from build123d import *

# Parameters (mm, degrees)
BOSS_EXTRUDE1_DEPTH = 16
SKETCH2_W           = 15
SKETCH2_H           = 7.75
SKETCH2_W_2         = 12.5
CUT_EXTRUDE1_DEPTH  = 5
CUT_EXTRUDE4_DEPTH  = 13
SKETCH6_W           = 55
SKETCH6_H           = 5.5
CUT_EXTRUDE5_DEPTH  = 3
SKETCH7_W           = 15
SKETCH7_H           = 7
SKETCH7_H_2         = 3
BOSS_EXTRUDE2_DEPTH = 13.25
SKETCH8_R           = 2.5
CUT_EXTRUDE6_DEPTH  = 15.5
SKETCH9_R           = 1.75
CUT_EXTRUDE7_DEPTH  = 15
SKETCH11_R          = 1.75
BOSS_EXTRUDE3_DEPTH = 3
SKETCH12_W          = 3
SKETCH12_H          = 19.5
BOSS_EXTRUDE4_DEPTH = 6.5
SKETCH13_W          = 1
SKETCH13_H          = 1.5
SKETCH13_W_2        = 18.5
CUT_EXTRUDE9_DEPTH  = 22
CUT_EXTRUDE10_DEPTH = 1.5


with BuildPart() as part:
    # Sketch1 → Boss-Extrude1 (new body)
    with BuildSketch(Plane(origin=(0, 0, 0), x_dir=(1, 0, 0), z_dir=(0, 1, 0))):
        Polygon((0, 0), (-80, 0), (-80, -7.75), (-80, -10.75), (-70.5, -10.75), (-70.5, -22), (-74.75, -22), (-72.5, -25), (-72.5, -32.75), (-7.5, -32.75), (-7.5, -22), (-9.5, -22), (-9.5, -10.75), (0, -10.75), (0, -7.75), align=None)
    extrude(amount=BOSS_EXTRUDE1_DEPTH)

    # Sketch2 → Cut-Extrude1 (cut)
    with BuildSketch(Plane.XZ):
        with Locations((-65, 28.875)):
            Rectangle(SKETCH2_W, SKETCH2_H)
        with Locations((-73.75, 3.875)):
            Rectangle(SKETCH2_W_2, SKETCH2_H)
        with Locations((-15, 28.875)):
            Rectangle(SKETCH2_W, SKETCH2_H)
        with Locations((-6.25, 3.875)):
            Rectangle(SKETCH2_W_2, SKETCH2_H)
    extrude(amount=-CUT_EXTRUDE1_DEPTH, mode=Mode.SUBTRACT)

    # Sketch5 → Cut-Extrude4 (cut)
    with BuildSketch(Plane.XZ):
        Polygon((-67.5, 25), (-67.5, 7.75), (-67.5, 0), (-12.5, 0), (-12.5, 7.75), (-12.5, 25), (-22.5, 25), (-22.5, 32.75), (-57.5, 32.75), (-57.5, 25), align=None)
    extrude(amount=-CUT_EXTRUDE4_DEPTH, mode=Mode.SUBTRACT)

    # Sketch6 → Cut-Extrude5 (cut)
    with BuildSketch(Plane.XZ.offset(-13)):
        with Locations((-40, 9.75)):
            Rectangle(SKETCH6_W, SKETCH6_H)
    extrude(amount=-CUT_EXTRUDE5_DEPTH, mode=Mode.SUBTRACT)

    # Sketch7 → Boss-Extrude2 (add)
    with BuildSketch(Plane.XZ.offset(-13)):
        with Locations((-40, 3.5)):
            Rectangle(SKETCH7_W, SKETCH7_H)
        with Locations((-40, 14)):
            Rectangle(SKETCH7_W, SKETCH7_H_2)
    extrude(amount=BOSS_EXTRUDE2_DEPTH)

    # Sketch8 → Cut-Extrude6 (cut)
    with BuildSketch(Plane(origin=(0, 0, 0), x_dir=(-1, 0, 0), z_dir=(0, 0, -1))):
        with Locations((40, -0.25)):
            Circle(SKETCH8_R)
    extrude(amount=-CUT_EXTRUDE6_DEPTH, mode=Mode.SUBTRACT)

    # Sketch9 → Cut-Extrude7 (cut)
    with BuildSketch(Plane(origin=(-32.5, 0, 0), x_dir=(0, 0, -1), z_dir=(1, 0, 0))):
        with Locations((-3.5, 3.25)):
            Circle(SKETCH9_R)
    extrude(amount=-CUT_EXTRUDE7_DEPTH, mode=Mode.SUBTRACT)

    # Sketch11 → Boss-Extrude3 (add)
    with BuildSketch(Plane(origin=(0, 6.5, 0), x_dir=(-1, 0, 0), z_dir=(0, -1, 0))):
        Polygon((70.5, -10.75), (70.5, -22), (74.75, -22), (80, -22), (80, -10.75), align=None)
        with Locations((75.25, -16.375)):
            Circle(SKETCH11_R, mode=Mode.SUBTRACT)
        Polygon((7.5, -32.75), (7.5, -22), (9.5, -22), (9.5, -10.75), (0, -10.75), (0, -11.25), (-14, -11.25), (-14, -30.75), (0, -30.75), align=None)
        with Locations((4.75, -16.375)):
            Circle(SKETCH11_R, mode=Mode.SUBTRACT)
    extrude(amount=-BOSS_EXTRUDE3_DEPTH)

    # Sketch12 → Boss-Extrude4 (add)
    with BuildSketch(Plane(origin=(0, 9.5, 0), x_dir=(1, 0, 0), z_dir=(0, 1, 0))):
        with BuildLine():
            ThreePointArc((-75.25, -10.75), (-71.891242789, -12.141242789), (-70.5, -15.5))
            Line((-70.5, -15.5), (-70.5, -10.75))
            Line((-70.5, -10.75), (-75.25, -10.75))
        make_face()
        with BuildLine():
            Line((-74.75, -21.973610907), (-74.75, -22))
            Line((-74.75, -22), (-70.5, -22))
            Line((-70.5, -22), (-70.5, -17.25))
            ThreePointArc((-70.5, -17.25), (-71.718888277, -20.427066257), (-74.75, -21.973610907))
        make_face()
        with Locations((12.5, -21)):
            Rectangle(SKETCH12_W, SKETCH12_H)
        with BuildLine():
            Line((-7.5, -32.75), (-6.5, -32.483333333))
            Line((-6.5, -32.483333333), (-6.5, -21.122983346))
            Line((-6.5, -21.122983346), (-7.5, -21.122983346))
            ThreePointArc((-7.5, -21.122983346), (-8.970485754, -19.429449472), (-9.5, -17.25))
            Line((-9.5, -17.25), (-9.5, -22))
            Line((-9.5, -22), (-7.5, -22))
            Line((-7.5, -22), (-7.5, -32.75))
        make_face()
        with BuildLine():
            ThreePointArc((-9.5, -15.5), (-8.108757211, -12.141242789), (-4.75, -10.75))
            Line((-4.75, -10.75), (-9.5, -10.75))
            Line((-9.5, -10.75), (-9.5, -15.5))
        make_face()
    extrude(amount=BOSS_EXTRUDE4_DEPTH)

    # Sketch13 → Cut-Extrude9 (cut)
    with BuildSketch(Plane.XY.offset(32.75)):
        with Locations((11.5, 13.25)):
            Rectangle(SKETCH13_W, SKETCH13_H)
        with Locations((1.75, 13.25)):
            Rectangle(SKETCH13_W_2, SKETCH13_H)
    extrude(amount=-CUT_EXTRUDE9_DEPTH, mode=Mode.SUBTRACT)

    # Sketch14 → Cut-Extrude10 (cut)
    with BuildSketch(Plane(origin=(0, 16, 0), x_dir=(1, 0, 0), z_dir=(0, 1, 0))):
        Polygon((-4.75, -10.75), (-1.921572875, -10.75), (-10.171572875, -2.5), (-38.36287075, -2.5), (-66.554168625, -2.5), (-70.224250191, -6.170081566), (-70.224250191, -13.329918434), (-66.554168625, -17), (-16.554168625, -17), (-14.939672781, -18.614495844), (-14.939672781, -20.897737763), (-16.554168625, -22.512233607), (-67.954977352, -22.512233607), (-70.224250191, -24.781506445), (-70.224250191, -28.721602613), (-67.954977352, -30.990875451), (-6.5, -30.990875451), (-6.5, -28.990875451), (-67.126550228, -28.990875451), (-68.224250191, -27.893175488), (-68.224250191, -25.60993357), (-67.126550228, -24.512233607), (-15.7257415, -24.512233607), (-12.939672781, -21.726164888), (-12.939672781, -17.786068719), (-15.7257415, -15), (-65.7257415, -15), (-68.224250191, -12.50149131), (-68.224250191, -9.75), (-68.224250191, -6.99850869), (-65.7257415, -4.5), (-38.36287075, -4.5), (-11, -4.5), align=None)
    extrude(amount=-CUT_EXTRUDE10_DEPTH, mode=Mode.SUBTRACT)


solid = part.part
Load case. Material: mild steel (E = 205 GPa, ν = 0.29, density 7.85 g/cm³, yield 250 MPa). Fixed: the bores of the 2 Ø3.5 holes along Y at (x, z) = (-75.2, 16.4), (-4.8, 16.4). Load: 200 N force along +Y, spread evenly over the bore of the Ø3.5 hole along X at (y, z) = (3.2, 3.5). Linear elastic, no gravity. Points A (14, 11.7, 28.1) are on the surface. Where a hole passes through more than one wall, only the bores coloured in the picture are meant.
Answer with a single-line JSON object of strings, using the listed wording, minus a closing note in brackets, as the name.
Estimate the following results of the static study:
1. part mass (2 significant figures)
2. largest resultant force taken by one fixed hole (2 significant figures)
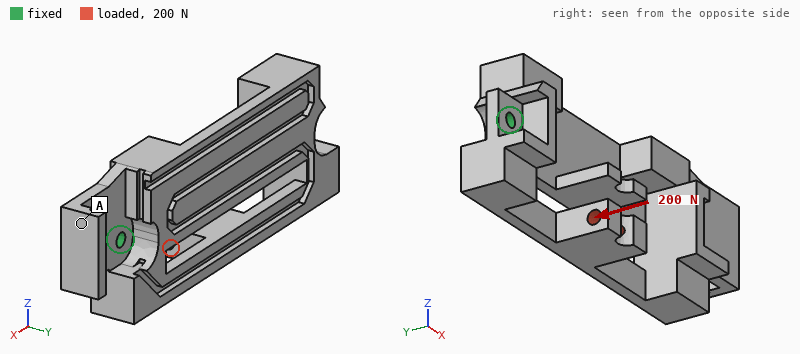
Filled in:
{"part mass": "120 g", "largest resultant force taken by one fixed hole": "210 N"}
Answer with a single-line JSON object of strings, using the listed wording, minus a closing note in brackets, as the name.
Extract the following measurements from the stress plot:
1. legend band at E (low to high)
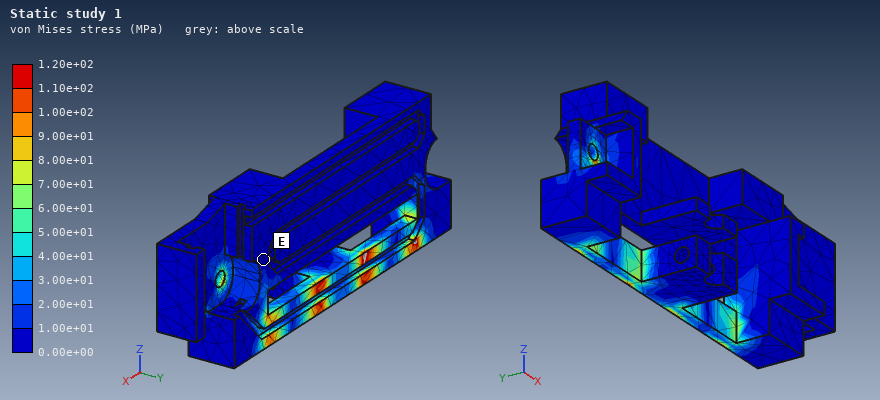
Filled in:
{"legend band at E": "0.00e+00 to 1.00e+01 MPa"}
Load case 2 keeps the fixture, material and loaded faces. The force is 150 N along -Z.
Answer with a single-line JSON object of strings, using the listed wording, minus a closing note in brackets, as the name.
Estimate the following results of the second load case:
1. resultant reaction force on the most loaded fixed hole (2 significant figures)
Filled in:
{"resultant reaction force on the most loaded fixed hole": "76 N"}
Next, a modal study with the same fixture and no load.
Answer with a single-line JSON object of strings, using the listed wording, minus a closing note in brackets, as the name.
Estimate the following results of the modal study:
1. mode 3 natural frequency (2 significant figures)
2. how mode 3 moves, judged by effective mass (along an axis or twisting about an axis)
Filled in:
{"mode 3 natural frequency": "3900 Hz", "how mode 3 moves, judged by effective mass": "along Y"}
